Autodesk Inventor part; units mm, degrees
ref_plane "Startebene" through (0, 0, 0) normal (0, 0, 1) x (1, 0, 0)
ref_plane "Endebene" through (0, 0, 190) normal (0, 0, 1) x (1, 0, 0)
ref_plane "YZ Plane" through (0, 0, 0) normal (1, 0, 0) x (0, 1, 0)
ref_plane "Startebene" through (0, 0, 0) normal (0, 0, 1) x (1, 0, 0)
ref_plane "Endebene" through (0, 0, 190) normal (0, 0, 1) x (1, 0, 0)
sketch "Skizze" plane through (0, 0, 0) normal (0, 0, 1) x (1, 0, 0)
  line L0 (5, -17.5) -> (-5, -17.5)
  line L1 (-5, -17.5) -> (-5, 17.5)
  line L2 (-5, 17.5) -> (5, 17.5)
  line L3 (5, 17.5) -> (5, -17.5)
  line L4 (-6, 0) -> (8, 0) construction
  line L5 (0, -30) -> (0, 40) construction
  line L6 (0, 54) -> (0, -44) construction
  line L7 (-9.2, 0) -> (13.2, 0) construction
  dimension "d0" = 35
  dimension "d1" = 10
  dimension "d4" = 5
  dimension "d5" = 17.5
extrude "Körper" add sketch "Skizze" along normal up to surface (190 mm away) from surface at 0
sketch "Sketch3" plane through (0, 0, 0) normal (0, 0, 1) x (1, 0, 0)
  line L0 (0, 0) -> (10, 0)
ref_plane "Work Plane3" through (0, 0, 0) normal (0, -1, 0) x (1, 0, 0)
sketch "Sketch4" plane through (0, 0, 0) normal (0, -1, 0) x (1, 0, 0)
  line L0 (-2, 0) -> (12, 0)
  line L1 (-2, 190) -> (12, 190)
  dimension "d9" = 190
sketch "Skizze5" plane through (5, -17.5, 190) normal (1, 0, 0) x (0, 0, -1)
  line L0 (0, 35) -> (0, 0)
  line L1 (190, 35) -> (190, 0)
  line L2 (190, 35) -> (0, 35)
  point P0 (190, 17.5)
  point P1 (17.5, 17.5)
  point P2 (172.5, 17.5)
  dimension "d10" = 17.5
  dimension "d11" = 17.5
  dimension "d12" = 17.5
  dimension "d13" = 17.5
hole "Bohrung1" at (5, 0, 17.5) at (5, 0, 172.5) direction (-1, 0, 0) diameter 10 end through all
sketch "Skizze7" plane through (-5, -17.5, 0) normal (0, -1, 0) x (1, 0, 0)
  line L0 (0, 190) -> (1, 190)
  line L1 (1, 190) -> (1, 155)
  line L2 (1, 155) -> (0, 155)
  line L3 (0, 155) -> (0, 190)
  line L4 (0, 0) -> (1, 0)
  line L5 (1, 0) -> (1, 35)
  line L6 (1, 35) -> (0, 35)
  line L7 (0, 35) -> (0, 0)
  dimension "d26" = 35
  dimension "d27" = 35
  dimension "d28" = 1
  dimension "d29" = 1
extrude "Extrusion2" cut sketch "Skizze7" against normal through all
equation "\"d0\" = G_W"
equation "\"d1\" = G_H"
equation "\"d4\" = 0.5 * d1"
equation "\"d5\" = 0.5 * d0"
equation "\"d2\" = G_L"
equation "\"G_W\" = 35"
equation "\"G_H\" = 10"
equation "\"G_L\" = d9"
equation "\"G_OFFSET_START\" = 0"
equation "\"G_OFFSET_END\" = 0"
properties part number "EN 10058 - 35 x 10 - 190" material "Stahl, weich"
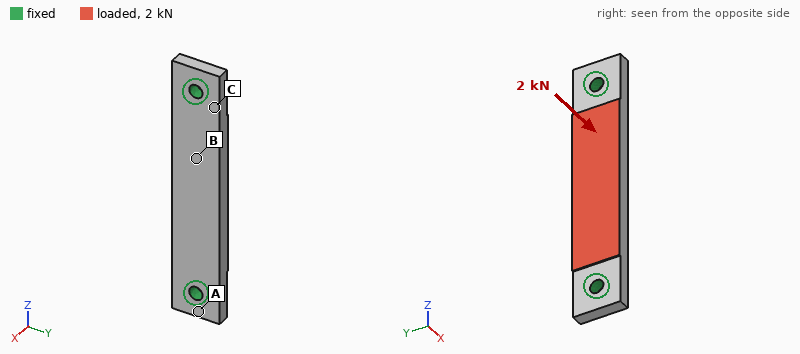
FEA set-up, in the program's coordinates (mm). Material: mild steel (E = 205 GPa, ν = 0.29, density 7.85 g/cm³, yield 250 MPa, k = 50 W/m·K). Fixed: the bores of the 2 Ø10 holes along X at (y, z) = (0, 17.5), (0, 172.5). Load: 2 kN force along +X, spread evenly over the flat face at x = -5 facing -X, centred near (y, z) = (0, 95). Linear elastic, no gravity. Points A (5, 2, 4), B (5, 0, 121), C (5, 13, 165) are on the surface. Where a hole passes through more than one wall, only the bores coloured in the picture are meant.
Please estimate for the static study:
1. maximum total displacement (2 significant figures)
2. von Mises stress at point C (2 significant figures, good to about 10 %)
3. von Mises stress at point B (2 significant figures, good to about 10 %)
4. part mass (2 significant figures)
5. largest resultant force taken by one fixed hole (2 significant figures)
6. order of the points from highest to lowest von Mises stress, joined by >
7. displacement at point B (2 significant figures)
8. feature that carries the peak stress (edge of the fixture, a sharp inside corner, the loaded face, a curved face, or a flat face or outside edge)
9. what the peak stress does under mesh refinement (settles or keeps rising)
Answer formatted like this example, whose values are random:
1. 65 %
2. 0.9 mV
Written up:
1. 46 µm
2. 32 MPa
3. 18 MPa
4. 490 g
5. 1.1 kN
6. C > B > A
7. 36 µm
8. edge of the fixture
9. keeps rising
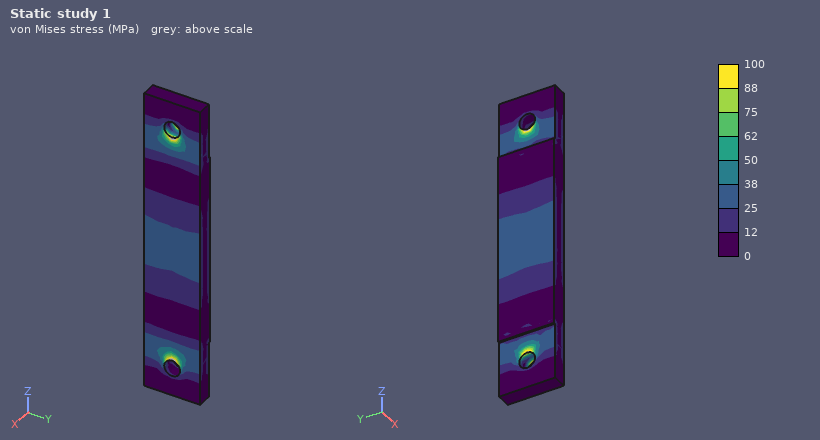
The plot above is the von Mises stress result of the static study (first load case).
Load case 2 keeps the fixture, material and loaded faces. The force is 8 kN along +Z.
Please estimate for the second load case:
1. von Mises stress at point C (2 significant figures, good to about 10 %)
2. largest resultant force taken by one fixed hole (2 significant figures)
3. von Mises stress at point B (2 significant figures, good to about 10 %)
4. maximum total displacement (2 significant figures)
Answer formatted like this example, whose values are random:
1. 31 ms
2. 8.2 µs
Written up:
1. 7.9 MPa
2. 4.0 kN
3. 4.6 MPa
4. 3.2 µm
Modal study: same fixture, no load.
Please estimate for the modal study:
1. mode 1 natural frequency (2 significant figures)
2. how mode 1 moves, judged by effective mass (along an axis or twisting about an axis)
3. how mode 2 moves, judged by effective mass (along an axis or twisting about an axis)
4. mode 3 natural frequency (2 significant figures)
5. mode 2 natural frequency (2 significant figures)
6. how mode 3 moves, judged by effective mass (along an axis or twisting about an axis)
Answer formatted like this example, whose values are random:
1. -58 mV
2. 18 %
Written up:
1. 2100 Hz
2. along X
3. along Y
4. 5100 Hz
5. 4700 Hz
6. twisting about Z
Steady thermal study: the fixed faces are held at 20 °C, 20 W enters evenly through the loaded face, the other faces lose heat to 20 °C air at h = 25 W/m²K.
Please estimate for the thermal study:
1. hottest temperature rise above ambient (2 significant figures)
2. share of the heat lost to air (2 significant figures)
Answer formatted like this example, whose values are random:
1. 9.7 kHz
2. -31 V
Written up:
1. 24 K
2. 18 %
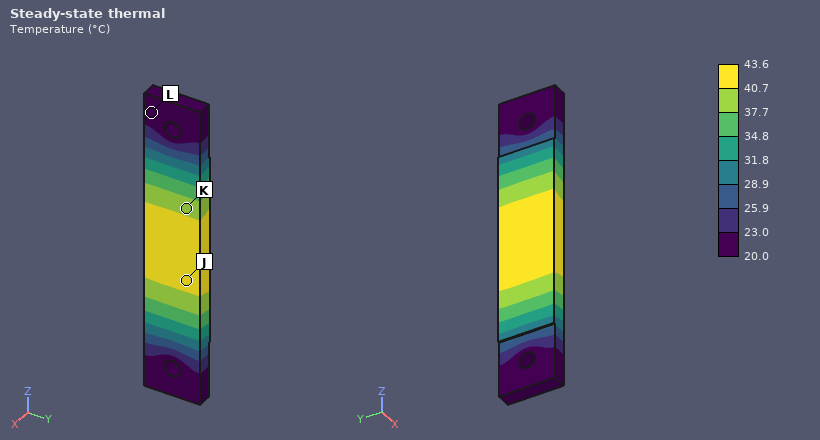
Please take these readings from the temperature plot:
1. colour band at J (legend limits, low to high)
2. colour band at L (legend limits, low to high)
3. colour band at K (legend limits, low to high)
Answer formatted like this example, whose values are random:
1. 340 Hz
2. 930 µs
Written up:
1. 40.7 to 43.6 °C
2. 20.0 to 23.0 °C
3. 37.7 to 40.7 °C
